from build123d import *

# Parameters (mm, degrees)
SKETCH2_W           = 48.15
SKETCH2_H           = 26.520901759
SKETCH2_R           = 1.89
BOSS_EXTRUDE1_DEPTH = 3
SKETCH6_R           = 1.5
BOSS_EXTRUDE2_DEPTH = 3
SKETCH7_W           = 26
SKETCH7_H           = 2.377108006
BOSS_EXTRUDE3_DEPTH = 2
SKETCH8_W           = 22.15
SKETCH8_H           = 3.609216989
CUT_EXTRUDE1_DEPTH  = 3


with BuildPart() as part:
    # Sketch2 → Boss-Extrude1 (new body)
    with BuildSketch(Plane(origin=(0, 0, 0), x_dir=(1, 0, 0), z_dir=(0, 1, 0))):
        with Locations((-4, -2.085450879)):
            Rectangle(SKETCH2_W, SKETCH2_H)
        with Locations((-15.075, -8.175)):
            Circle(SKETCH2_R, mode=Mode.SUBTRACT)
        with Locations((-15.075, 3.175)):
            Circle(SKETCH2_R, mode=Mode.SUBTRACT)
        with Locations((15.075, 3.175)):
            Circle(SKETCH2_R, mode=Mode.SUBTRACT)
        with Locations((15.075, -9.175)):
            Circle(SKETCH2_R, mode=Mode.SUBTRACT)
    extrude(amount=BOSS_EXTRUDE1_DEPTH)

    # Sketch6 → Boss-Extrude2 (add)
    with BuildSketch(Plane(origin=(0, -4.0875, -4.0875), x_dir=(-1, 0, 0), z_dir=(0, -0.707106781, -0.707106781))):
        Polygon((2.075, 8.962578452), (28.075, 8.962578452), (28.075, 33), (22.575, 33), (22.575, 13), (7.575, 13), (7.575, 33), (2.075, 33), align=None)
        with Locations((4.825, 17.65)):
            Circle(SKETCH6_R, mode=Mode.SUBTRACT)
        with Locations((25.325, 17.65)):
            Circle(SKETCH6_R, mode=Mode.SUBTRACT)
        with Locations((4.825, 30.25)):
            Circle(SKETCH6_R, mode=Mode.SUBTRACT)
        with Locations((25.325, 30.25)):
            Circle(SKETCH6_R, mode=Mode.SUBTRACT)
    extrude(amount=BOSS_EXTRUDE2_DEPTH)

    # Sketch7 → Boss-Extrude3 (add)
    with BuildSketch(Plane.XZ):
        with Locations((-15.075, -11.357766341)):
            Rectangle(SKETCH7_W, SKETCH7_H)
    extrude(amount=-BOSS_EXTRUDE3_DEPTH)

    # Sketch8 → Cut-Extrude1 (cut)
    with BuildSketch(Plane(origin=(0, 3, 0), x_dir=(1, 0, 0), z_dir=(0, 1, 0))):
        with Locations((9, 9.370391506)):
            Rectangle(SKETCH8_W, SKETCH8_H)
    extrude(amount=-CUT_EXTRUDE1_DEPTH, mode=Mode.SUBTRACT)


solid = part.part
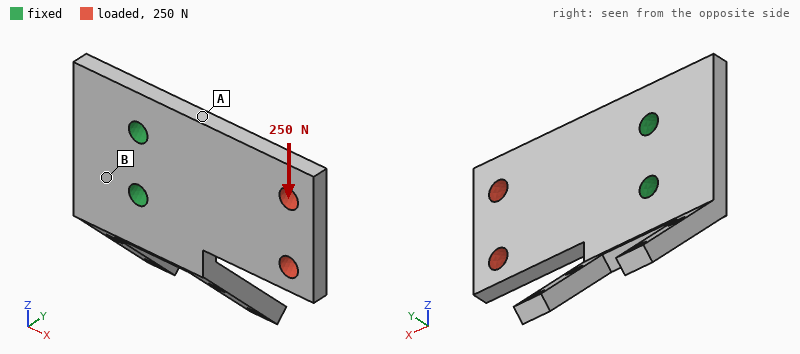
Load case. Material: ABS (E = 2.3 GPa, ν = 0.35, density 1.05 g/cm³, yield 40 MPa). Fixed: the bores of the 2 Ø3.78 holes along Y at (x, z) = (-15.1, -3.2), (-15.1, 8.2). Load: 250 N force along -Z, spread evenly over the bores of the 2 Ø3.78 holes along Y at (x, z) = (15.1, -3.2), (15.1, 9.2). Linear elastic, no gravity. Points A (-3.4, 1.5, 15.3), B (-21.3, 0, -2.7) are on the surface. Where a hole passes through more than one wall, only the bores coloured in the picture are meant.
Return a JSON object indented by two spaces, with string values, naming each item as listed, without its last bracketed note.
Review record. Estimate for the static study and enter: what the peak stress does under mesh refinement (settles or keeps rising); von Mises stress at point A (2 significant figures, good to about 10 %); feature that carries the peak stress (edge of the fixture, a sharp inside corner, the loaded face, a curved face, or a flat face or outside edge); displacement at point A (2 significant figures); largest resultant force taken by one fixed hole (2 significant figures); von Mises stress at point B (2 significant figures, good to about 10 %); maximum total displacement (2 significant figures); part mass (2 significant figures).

{
  "what the peak stress does under mesh refinement": "keeps rising",
  "von Mises stress at point A": "15 MPa",
  "feature that carries the peak stress": "edge of the fixture",
  "displacement at point A": "0.20 mm",
  "largest resultant force taken by one fixed hole": "560 N",
  "von Mises stress at point B": "5.0 MPa",
  "maximum total displacement": "0.61 mm",
  "part mass": "4.6 g"
}
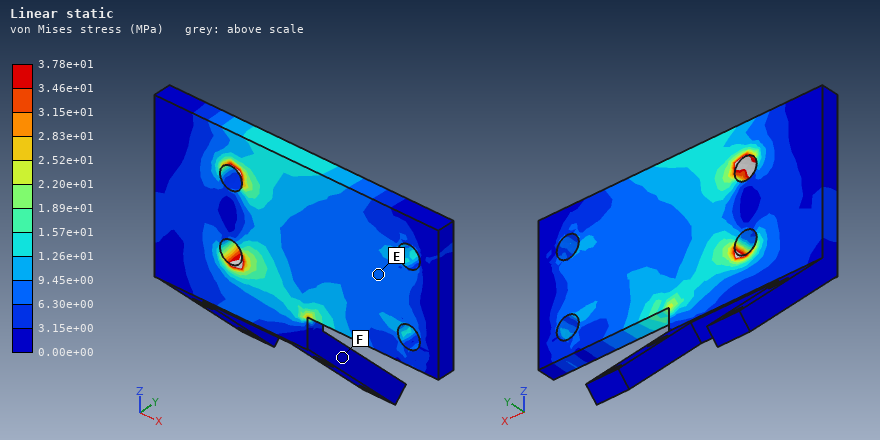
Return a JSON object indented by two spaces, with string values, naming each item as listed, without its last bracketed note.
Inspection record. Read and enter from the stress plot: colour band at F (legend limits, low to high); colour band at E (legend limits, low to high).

{
  "colour band at F": "0.00e+00 to 3.15e+00 MPa",
  "colour band at E": "6.30e+00 to 9.45e+00 MPa"
}
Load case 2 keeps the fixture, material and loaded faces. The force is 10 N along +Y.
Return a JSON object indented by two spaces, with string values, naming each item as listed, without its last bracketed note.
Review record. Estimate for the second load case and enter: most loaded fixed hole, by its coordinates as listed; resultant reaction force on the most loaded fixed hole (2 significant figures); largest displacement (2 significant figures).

{
  "most loaded fixed hole, by its coordinates as listed": "(-15.1, 8.2)",
  "resultant reaction force on the most loaded fixed hole": "5.9 N",
  "largest displacement": "0.77 mm"
}
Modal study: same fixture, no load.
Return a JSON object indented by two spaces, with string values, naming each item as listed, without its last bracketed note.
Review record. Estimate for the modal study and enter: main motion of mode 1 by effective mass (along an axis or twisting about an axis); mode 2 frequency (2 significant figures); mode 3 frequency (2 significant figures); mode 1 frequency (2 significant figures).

{
  "main motion of mode 1 by effective mass": "along Y",
  "mode 2 frequency": "970 Hz",
  "mode 3 frequency": "1000 Hz",
  "mode 1 frequency": "680 Hz"
}
